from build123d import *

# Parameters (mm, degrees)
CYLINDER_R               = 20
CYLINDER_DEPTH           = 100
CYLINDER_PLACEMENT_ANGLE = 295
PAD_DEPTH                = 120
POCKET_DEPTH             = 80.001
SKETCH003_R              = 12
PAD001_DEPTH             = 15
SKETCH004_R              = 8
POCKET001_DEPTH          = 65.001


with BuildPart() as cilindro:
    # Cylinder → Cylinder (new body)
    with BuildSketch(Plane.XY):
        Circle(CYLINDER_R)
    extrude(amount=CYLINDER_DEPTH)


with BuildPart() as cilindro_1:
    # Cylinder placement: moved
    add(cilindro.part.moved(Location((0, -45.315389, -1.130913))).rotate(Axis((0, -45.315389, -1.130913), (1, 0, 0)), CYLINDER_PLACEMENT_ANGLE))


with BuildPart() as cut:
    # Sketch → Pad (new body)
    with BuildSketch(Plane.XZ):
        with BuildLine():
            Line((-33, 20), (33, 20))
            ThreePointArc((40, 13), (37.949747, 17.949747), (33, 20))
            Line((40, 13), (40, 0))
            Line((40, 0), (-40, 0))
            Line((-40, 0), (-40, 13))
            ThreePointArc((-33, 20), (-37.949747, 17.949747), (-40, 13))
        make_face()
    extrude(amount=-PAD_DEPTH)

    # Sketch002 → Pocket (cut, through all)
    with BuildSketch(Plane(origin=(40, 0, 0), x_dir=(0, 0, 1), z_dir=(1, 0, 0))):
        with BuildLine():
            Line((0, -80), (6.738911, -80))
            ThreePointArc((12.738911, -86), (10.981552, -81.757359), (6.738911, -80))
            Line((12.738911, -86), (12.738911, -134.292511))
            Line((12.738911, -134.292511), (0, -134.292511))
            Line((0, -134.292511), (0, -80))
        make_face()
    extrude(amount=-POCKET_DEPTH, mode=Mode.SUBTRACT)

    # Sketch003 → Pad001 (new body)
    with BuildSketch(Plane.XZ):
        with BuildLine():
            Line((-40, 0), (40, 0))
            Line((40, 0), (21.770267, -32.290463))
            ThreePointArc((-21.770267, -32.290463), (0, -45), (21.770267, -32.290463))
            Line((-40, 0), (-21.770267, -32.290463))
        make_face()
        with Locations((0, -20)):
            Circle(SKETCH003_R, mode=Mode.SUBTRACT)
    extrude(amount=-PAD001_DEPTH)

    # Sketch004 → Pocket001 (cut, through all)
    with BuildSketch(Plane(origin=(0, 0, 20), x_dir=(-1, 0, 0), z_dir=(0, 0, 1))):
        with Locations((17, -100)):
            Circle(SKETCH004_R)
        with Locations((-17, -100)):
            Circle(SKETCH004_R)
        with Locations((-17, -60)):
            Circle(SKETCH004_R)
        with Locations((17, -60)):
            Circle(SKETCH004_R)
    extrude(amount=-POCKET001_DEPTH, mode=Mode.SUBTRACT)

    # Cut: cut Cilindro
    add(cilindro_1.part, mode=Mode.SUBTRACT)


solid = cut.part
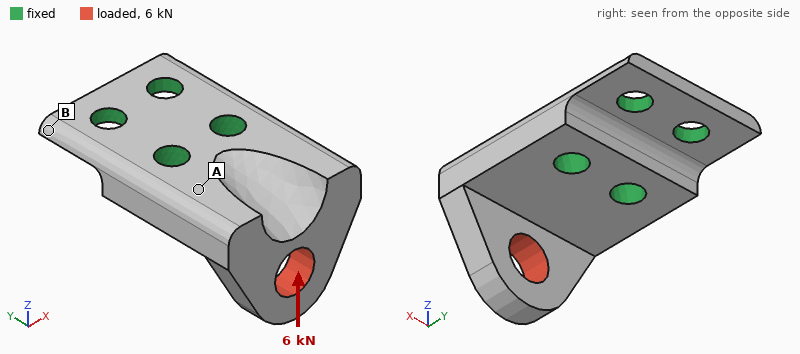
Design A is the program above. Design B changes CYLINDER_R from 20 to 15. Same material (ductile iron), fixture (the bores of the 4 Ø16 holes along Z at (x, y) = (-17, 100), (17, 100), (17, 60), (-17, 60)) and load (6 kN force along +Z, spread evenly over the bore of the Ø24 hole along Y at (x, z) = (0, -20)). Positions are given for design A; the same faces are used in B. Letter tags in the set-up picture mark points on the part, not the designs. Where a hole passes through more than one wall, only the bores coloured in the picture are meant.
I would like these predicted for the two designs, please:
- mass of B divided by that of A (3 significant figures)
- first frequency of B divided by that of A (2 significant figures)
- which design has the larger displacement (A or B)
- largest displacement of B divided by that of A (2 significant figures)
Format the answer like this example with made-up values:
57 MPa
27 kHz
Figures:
1.05
1.0
A
0.89
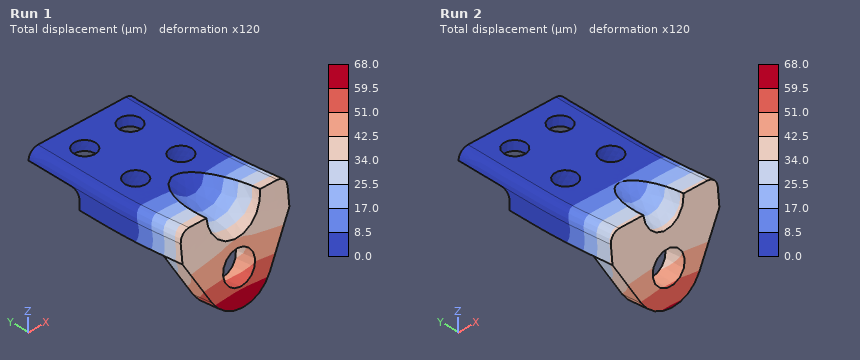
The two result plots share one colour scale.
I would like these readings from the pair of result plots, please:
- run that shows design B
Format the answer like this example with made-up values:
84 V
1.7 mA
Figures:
Run 2
